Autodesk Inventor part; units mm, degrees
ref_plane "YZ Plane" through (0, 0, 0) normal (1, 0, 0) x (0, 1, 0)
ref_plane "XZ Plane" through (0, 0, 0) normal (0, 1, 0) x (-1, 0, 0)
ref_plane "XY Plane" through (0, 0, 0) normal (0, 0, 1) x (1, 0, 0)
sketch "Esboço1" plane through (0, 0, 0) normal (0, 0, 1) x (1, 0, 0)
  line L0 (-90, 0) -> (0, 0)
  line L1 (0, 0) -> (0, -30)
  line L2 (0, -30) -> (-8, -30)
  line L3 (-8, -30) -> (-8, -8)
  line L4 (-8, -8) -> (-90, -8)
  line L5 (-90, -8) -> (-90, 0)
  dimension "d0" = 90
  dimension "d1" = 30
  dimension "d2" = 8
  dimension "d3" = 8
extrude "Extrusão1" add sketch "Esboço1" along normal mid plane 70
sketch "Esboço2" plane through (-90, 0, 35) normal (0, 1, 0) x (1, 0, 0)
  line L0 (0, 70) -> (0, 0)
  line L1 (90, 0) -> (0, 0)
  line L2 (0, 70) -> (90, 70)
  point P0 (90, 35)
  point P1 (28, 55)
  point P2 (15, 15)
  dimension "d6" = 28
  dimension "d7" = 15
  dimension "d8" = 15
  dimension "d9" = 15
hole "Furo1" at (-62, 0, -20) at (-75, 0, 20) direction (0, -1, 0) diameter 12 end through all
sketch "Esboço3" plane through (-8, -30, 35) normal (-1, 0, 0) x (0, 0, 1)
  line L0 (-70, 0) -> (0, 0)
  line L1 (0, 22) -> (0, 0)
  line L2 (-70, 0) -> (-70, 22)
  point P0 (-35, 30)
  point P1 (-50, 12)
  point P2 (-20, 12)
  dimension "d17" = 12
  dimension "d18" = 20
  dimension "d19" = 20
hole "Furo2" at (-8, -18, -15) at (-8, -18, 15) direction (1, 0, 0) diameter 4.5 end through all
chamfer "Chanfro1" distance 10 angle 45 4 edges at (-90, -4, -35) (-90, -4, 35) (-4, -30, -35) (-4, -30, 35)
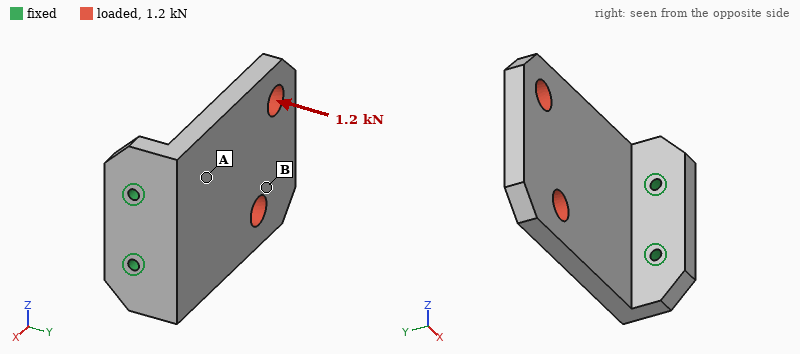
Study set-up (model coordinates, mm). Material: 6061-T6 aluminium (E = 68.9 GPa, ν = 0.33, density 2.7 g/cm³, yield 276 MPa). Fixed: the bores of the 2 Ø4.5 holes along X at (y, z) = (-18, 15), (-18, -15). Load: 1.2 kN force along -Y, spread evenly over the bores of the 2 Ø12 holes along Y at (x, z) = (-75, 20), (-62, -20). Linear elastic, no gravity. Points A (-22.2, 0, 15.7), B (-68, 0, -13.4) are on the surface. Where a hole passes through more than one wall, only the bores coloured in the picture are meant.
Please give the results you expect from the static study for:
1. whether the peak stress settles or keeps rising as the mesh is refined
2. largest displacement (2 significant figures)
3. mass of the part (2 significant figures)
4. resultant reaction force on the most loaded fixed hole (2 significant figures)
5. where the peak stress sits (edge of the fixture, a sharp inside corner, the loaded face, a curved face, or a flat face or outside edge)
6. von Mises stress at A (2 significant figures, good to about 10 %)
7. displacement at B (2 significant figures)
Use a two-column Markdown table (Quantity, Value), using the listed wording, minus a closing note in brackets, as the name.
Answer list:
| Quantity | Value |
|---|---|
| whether the peak stress settles or keeps rising as the mesh is refined | keeps rising |
| largest displacement | 1.2 mm |
| mass of the part | 160 g |
| resultant reaction force on the most loaded fixed hole | 640 N |
| where the peak stress sits | edge of the fixture |
| von Mises stress at A | 68 MPa |
| displacement at B | 0.85 mm |
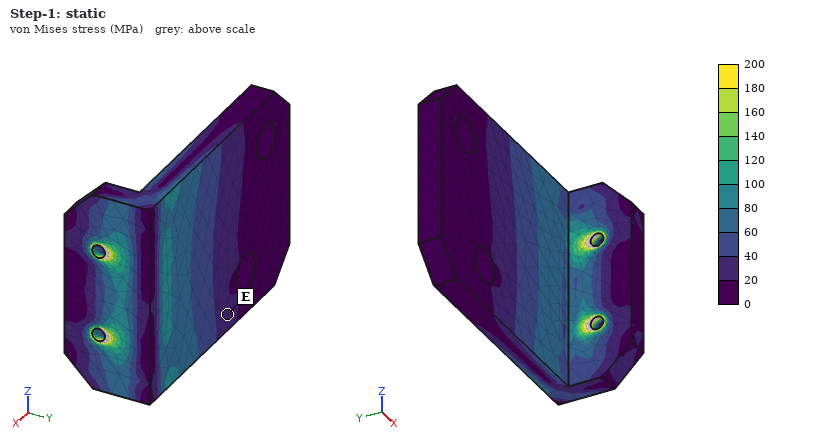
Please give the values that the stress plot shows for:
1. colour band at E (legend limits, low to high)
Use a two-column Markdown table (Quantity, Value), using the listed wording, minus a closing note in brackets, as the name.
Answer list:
| Quantity | Value |
|---|---|
| colour band at E | 20 to 40 MPa |
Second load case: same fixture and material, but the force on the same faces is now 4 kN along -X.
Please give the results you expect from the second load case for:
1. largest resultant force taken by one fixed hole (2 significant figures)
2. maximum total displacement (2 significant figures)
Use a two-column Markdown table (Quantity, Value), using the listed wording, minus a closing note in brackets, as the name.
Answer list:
| Quantity | Value |
|---|---|
| largest resultant force taken by one fixed hole | 2.0 kN |
| maximum total displacement | 0.26 mm |
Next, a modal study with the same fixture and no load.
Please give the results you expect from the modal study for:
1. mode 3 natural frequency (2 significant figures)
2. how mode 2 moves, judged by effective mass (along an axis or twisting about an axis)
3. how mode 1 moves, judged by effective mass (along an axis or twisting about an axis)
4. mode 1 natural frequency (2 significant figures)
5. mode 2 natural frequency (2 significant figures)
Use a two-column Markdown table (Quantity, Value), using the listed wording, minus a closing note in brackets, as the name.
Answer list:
| Quantity | Value |
|---|---|
| mode 3 natural frequency | 2600 Hz |
| how mode 2 moves, judged by effective mass | along Z |
| how mode 1 moves, judged by effective mass | along Y |
| mode 1 natural frequency | 730 Hz |
| mode 2 natural frequency | 1900 Hz |
